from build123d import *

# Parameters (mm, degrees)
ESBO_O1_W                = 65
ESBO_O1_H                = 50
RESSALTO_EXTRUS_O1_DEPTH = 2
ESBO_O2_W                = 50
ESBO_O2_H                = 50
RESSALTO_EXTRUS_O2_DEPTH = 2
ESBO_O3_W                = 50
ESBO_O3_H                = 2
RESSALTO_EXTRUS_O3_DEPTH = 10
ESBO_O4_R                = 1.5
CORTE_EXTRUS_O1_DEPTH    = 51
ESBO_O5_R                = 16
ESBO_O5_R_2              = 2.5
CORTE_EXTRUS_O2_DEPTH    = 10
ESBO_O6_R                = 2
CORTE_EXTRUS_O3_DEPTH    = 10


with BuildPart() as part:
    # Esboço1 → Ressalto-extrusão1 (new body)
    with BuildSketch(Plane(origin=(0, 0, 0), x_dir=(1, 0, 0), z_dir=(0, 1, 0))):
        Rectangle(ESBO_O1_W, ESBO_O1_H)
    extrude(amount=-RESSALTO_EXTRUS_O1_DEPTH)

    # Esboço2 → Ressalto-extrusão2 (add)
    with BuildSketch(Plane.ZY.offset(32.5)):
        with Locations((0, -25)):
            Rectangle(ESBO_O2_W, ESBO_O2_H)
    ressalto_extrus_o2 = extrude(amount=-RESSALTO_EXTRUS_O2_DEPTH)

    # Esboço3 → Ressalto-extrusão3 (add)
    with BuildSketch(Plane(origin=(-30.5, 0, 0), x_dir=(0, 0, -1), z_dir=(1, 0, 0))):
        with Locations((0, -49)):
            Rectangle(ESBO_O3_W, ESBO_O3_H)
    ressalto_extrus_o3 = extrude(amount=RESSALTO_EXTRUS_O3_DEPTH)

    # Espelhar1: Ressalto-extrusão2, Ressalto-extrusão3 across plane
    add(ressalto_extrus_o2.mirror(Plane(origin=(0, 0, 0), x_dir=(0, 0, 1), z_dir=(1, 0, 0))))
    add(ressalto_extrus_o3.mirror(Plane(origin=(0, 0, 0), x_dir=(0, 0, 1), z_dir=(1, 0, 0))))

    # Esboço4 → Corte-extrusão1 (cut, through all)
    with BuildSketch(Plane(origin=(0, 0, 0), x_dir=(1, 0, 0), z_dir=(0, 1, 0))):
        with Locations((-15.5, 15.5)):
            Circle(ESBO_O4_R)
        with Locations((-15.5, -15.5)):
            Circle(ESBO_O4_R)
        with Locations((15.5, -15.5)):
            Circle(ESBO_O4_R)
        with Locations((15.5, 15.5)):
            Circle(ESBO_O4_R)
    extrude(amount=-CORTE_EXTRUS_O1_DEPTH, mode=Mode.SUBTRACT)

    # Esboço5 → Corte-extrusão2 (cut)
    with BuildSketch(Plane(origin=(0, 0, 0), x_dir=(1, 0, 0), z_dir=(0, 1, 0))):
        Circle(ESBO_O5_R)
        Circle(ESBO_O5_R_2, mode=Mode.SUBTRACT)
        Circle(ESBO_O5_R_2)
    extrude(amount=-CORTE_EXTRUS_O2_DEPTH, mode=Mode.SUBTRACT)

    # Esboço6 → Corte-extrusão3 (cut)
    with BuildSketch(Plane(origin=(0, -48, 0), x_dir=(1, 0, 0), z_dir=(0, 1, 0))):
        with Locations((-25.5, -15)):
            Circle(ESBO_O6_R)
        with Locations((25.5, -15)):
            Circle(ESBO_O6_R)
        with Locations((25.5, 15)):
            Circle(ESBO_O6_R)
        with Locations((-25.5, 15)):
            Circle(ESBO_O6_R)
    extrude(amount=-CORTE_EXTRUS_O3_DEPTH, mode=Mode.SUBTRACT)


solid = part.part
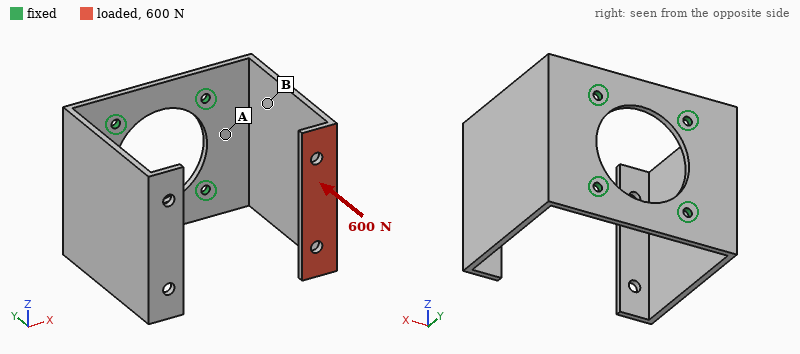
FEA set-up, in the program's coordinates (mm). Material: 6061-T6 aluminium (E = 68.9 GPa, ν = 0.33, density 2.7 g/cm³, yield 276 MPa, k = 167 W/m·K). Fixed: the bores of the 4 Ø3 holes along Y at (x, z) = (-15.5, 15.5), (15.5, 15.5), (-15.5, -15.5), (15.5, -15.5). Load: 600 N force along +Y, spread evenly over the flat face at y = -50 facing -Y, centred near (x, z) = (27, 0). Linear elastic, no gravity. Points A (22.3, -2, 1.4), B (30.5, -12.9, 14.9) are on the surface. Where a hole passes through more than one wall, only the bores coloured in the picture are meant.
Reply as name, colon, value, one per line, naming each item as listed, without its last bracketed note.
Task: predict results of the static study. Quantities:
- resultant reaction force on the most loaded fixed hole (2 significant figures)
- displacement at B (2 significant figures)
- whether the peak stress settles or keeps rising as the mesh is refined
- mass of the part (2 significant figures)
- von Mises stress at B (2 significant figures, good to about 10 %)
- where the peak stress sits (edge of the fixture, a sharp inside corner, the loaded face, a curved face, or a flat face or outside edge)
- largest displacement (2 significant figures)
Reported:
resultant reaction force on the most loaded fixed hole: 310 N
displacement at B: 0.28 mm
whether the peak stress settles or keeps rising as the mesh is refined: keeps rising
mass of the part: 44 g
von Mises stress at B: 89 MPa
where the peak stress sits: edge of the fixture
largest displacement: 0.93 mm
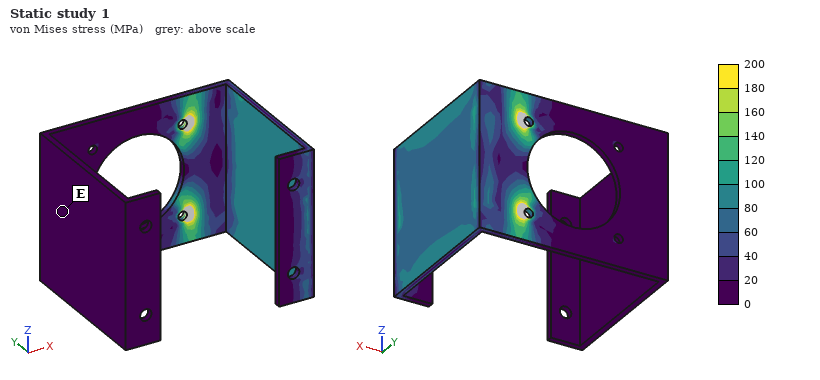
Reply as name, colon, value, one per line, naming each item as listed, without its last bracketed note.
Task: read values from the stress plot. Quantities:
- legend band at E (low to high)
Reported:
legend band at E: 0 to 20 MPa
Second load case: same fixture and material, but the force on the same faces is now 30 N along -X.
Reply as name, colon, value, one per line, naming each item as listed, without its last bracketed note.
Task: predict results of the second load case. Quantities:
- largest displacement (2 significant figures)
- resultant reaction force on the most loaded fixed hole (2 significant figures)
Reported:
largest displacement: 0.98 mm
resultant reaction force on the most loaded fixed hole: 21 N
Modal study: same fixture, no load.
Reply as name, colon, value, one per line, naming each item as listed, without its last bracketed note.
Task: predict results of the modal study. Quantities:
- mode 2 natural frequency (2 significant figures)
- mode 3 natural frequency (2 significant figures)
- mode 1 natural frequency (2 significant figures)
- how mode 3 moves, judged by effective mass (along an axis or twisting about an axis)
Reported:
mode 2 natural frequency: 350 Hz
mode 3 natural frequency: 890 Hz
mode 1 natural frequency: 350 Hz
how mode 3 moves, judged by effective mass: along Z
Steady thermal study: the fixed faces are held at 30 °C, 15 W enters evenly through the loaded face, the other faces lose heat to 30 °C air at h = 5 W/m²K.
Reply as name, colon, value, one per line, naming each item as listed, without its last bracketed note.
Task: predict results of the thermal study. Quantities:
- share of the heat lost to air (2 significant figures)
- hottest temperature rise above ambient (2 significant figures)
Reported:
share of the heat lost to air: 8.1 %
hottest temperature rise above ambient: 62 K
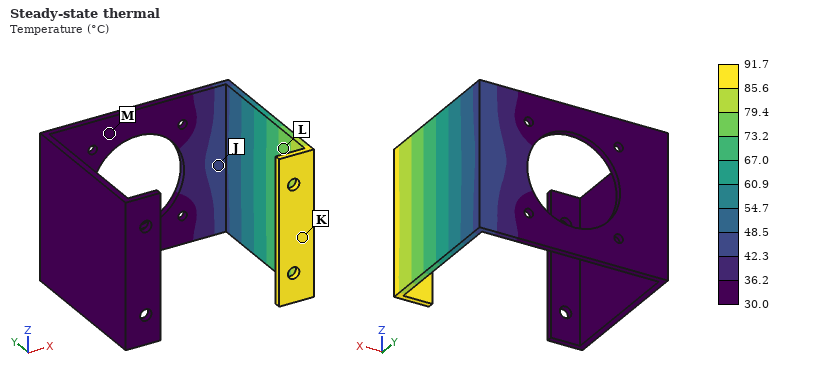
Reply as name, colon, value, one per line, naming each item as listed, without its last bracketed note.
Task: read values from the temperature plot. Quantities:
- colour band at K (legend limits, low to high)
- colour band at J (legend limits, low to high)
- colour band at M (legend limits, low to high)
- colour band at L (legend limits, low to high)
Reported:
colour band at K: 85.6 to 91.7 °C
colour band at J: 42.3 to 48.5 °C
colour band at M: 30.0 to 36.2 °C
colour band at L: 73.2 to 79.4 °C
